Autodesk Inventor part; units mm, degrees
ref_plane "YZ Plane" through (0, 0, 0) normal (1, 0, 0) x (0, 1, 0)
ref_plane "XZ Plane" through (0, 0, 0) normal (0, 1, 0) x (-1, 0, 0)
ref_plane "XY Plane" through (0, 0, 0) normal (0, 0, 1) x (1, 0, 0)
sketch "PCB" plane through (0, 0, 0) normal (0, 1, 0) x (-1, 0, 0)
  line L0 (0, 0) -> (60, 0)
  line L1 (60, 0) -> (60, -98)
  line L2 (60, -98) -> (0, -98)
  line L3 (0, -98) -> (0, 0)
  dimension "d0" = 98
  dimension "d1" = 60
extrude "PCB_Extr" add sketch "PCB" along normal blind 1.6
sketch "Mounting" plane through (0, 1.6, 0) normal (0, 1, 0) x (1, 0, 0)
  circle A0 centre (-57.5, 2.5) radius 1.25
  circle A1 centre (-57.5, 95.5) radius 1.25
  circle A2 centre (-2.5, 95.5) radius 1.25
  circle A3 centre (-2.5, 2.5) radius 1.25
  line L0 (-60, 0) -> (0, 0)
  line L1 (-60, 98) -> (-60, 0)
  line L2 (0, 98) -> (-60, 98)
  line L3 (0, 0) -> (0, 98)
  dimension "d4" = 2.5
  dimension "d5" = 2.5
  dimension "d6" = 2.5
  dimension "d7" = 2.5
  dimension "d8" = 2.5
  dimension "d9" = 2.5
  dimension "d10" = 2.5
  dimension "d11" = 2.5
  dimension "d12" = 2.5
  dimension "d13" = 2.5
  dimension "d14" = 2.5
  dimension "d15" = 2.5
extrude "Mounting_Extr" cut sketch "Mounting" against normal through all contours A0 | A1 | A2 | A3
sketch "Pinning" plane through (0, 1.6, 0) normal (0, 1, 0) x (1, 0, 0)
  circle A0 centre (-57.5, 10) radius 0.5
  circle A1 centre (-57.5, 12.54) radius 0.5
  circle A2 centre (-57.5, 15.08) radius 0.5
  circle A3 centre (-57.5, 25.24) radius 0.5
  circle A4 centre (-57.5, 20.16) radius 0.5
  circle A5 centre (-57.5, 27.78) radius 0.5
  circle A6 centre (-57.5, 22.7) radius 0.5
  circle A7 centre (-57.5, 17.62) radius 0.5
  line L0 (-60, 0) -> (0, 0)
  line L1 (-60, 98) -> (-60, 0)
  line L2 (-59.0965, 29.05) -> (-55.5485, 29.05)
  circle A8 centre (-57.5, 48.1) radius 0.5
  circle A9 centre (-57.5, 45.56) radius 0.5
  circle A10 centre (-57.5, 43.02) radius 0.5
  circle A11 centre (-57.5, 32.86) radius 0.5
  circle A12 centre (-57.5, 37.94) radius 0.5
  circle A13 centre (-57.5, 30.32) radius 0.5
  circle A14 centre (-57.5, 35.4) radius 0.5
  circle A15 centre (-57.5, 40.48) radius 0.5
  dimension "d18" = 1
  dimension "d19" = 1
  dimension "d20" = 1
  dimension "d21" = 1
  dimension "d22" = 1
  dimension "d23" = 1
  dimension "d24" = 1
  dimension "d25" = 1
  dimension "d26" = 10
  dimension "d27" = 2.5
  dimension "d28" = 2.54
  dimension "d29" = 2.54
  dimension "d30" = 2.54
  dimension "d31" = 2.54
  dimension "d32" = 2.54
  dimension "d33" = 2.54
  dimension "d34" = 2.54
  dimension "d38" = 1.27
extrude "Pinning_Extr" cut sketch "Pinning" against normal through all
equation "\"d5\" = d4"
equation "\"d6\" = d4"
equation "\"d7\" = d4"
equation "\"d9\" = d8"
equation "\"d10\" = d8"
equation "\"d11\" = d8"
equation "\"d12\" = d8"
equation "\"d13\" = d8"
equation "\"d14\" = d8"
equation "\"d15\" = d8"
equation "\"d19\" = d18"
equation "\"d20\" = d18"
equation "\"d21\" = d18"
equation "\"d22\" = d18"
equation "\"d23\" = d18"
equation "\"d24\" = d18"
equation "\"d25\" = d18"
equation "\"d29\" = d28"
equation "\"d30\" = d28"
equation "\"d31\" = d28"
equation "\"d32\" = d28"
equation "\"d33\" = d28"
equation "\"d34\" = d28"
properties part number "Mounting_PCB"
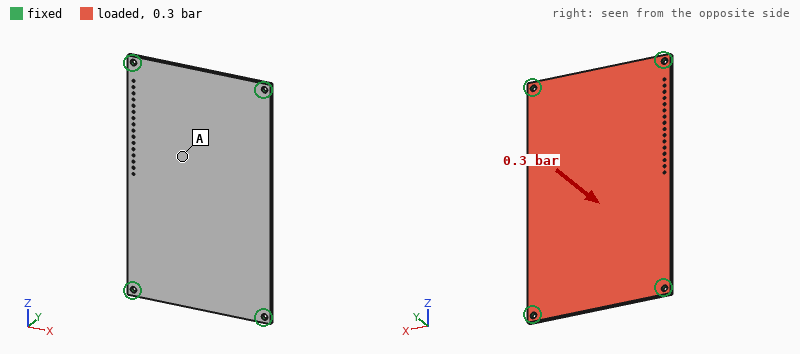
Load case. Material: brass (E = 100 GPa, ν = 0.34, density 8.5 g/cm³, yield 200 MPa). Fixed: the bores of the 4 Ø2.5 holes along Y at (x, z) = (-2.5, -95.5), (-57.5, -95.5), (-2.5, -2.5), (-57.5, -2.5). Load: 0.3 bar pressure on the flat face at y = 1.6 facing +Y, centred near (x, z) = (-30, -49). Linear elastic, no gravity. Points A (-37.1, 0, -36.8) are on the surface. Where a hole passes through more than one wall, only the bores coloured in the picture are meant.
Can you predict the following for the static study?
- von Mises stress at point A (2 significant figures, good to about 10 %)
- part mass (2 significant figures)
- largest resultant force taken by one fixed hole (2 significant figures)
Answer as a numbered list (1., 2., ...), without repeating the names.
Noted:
1. 25 MPa
2. 80 g
3. 44 N
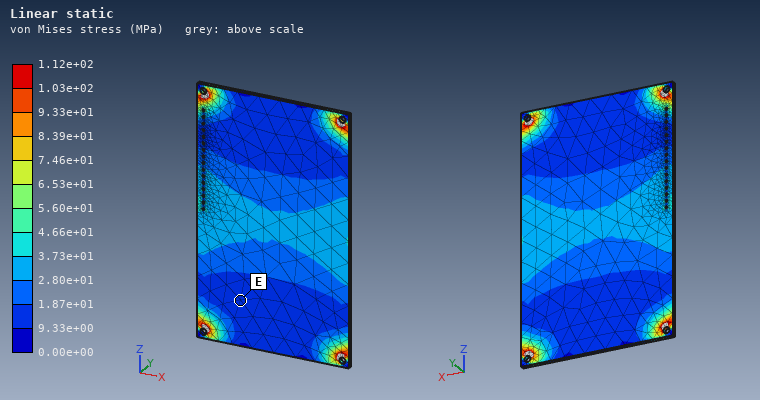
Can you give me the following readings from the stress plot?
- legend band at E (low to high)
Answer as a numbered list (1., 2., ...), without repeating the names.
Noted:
1. 9.33e+00 to 1.87e+01 MPa
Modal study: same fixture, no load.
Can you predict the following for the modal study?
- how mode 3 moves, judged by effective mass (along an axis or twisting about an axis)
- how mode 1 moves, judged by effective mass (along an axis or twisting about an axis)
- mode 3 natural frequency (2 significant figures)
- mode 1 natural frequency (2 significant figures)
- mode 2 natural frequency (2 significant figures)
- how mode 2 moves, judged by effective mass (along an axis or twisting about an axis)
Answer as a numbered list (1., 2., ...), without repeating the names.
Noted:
1. twisting about X
2. along Y
3. 1400 Hz
4. 510 Hz
5. 910 Hz
6. twisting about Z
